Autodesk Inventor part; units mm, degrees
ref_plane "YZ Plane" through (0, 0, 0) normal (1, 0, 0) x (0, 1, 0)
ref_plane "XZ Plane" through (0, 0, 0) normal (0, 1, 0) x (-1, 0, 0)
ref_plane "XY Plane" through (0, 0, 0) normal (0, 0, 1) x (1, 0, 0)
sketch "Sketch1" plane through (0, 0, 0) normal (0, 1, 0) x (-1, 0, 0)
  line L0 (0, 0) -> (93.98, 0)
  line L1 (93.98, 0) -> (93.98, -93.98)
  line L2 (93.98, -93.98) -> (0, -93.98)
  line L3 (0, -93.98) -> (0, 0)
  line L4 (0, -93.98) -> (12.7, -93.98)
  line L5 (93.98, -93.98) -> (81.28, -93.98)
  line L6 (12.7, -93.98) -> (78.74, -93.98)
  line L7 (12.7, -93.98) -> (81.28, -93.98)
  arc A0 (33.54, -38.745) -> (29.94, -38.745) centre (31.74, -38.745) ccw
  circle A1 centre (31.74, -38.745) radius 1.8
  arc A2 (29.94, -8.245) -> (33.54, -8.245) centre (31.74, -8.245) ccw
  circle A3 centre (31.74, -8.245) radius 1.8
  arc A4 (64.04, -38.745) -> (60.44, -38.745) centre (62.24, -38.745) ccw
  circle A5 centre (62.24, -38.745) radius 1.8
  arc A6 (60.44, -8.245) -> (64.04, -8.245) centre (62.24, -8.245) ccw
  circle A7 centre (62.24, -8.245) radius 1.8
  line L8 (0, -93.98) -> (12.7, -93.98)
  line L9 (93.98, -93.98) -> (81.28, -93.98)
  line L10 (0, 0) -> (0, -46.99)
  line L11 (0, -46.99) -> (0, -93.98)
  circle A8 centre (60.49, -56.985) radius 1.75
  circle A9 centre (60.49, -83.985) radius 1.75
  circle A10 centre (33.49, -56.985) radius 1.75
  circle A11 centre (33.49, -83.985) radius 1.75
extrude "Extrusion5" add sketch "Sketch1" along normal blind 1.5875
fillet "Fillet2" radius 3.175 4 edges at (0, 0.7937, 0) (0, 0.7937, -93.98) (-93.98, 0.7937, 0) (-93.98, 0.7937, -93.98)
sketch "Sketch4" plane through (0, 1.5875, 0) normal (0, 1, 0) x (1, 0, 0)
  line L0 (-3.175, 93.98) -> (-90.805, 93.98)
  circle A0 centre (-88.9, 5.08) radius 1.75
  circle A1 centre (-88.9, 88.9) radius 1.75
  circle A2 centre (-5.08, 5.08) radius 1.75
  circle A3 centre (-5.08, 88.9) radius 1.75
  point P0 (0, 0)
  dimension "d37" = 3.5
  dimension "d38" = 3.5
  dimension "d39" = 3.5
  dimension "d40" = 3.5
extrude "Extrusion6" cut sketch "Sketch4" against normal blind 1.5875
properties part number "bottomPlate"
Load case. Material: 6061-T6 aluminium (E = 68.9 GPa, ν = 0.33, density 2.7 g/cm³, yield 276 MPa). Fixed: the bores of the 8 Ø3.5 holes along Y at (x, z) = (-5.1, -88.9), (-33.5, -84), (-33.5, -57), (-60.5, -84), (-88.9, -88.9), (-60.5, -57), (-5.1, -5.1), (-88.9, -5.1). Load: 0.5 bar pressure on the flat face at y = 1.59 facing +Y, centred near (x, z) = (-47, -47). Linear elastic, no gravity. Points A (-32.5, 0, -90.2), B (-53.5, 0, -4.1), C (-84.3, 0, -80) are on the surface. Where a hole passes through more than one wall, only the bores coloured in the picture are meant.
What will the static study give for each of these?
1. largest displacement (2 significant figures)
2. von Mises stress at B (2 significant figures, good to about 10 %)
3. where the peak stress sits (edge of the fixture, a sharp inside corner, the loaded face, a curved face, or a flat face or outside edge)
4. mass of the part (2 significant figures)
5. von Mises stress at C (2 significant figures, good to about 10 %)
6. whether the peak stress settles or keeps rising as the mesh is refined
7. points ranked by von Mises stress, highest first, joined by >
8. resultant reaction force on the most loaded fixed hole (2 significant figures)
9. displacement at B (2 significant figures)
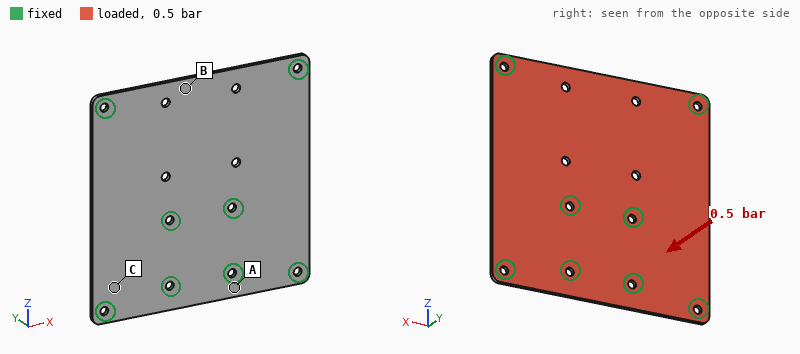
0.25 mm
26 MPa
edge of the fixture
37 g
13 MPa
keeps rising
B > C > A
96 N
0.23 mm
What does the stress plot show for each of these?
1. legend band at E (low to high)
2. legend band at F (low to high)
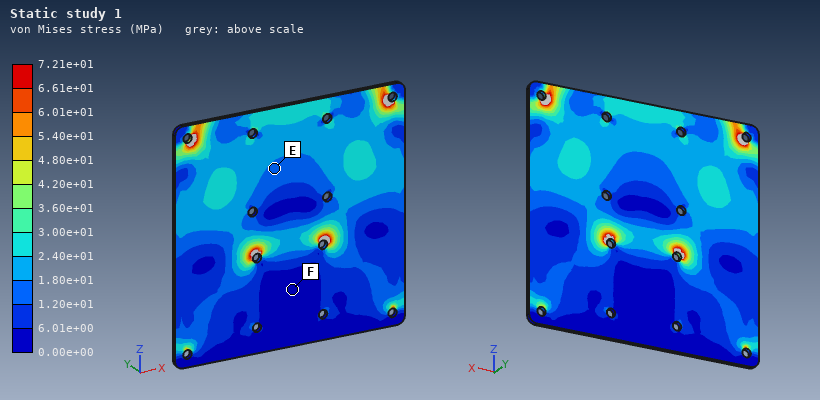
1.20e+01 to 1.80e+01 MPa
0.00e+00 to 6.01e+00 MPa
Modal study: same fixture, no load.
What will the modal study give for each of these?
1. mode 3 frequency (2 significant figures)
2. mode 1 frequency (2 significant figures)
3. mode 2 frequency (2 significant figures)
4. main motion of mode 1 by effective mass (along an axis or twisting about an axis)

1900 Hz
1300 Hz
1900 Hz
along Y
